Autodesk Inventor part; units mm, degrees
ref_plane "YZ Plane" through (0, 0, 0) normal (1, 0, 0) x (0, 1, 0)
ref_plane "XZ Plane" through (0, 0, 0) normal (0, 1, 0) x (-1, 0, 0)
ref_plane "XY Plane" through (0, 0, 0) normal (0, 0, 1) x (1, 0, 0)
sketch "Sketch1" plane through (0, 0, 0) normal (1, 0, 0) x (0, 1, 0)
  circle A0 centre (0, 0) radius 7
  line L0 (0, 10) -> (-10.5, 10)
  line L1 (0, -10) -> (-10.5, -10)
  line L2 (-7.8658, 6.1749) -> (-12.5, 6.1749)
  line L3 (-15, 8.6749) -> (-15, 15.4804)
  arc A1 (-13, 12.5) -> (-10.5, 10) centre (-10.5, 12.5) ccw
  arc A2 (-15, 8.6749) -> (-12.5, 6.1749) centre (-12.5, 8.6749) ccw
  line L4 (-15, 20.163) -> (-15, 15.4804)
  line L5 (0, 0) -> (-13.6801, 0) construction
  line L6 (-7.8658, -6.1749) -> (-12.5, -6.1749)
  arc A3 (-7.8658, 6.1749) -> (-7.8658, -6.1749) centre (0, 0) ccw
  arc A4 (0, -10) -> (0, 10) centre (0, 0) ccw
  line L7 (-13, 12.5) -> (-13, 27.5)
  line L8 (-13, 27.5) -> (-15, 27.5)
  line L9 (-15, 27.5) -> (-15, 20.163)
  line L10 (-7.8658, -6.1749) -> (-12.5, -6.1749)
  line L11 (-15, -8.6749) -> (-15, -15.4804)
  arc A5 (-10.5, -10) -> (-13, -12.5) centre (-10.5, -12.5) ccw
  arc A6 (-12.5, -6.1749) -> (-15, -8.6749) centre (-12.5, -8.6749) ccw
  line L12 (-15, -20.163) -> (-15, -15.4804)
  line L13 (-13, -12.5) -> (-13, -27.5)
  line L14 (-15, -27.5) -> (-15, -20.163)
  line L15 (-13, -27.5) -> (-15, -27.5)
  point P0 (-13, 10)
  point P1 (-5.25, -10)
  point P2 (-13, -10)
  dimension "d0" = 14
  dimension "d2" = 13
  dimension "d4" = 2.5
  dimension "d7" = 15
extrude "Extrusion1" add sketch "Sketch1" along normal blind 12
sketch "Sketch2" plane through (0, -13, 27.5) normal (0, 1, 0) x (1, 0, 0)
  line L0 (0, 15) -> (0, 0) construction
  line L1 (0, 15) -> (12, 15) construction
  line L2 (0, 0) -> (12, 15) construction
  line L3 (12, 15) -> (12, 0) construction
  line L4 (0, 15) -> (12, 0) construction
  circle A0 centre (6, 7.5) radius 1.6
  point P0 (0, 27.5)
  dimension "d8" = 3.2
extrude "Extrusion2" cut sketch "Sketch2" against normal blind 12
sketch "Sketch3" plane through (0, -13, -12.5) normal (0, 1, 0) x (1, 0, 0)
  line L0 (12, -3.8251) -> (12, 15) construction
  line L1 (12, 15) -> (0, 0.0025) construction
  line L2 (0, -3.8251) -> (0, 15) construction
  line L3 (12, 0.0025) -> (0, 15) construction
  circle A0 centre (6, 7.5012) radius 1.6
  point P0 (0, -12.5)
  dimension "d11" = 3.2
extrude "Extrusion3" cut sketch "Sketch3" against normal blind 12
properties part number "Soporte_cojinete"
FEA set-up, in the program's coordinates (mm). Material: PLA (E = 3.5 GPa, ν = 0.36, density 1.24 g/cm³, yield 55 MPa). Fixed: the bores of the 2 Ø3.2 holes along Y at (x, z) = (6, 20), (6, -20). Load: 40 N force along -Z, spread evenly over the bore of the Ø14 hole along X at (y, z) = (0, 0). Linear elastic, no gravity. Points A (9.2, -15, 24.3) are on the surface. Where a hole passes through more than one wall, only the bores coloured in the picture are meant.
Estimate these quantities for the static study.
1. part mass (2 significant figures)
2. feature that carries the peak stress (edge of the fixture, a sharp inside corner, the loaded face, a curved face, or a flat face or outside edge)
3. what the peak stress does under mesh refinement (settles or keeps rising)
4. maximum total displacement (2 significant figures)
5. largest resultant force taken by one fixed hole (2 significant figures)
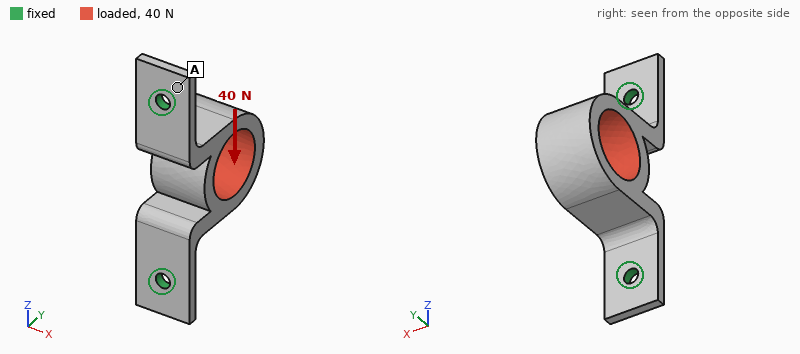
4.5 g
edge of the fixture
keeps rising
0.10 mm
27 N
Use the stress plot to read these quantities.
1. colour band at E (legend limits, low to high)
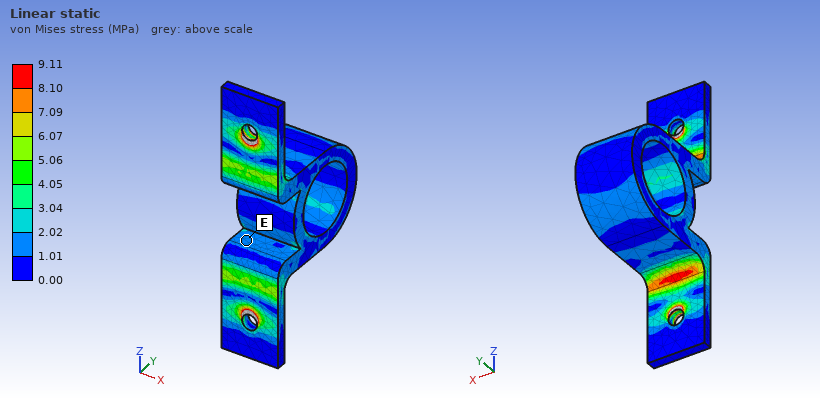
1.01 to 2.02 MPa
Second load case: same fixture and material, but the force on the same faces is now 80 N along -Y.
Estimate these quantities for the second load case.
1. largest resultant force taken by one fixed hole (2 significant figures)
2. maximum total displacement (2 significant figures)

57 N
0.12 mm
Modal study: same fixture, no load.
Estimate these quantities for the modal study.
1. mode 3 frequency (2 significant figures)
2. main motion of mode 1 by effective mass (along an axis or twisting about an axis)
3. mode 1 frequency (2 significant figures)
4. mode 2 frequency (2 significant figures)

2200 Hz
along X
670 Hz
2100 Hz
